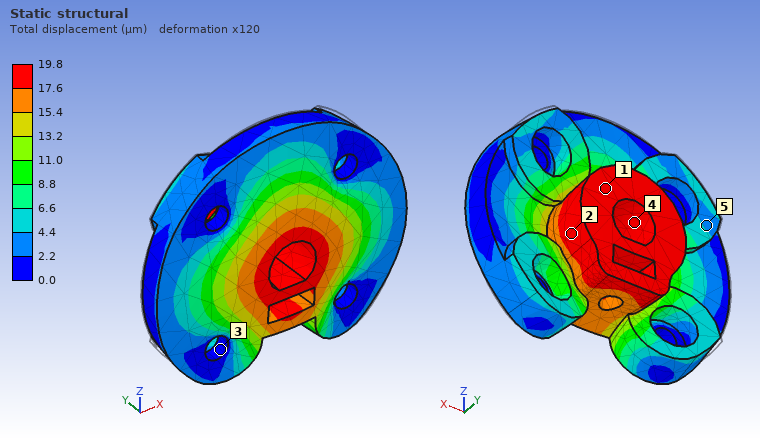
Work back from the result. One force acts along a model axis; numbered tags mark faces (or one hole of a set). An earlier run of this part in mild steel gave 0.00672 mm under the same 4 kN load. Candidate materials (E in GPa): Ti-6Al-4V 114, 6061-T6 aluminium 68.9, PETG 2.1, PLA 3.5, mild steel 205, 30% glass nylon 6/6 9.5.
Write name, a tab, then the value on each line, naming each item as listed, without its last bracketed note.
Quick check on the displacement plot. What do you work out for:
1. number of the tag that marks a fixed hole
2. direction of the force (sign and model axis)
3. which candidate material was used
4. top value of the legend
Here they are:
number of the tag that marks a fixed hole	3
direction of the force	-Y
which candidate material was used	6061-T6 aluminium
top value of the legend	19.8 µm
